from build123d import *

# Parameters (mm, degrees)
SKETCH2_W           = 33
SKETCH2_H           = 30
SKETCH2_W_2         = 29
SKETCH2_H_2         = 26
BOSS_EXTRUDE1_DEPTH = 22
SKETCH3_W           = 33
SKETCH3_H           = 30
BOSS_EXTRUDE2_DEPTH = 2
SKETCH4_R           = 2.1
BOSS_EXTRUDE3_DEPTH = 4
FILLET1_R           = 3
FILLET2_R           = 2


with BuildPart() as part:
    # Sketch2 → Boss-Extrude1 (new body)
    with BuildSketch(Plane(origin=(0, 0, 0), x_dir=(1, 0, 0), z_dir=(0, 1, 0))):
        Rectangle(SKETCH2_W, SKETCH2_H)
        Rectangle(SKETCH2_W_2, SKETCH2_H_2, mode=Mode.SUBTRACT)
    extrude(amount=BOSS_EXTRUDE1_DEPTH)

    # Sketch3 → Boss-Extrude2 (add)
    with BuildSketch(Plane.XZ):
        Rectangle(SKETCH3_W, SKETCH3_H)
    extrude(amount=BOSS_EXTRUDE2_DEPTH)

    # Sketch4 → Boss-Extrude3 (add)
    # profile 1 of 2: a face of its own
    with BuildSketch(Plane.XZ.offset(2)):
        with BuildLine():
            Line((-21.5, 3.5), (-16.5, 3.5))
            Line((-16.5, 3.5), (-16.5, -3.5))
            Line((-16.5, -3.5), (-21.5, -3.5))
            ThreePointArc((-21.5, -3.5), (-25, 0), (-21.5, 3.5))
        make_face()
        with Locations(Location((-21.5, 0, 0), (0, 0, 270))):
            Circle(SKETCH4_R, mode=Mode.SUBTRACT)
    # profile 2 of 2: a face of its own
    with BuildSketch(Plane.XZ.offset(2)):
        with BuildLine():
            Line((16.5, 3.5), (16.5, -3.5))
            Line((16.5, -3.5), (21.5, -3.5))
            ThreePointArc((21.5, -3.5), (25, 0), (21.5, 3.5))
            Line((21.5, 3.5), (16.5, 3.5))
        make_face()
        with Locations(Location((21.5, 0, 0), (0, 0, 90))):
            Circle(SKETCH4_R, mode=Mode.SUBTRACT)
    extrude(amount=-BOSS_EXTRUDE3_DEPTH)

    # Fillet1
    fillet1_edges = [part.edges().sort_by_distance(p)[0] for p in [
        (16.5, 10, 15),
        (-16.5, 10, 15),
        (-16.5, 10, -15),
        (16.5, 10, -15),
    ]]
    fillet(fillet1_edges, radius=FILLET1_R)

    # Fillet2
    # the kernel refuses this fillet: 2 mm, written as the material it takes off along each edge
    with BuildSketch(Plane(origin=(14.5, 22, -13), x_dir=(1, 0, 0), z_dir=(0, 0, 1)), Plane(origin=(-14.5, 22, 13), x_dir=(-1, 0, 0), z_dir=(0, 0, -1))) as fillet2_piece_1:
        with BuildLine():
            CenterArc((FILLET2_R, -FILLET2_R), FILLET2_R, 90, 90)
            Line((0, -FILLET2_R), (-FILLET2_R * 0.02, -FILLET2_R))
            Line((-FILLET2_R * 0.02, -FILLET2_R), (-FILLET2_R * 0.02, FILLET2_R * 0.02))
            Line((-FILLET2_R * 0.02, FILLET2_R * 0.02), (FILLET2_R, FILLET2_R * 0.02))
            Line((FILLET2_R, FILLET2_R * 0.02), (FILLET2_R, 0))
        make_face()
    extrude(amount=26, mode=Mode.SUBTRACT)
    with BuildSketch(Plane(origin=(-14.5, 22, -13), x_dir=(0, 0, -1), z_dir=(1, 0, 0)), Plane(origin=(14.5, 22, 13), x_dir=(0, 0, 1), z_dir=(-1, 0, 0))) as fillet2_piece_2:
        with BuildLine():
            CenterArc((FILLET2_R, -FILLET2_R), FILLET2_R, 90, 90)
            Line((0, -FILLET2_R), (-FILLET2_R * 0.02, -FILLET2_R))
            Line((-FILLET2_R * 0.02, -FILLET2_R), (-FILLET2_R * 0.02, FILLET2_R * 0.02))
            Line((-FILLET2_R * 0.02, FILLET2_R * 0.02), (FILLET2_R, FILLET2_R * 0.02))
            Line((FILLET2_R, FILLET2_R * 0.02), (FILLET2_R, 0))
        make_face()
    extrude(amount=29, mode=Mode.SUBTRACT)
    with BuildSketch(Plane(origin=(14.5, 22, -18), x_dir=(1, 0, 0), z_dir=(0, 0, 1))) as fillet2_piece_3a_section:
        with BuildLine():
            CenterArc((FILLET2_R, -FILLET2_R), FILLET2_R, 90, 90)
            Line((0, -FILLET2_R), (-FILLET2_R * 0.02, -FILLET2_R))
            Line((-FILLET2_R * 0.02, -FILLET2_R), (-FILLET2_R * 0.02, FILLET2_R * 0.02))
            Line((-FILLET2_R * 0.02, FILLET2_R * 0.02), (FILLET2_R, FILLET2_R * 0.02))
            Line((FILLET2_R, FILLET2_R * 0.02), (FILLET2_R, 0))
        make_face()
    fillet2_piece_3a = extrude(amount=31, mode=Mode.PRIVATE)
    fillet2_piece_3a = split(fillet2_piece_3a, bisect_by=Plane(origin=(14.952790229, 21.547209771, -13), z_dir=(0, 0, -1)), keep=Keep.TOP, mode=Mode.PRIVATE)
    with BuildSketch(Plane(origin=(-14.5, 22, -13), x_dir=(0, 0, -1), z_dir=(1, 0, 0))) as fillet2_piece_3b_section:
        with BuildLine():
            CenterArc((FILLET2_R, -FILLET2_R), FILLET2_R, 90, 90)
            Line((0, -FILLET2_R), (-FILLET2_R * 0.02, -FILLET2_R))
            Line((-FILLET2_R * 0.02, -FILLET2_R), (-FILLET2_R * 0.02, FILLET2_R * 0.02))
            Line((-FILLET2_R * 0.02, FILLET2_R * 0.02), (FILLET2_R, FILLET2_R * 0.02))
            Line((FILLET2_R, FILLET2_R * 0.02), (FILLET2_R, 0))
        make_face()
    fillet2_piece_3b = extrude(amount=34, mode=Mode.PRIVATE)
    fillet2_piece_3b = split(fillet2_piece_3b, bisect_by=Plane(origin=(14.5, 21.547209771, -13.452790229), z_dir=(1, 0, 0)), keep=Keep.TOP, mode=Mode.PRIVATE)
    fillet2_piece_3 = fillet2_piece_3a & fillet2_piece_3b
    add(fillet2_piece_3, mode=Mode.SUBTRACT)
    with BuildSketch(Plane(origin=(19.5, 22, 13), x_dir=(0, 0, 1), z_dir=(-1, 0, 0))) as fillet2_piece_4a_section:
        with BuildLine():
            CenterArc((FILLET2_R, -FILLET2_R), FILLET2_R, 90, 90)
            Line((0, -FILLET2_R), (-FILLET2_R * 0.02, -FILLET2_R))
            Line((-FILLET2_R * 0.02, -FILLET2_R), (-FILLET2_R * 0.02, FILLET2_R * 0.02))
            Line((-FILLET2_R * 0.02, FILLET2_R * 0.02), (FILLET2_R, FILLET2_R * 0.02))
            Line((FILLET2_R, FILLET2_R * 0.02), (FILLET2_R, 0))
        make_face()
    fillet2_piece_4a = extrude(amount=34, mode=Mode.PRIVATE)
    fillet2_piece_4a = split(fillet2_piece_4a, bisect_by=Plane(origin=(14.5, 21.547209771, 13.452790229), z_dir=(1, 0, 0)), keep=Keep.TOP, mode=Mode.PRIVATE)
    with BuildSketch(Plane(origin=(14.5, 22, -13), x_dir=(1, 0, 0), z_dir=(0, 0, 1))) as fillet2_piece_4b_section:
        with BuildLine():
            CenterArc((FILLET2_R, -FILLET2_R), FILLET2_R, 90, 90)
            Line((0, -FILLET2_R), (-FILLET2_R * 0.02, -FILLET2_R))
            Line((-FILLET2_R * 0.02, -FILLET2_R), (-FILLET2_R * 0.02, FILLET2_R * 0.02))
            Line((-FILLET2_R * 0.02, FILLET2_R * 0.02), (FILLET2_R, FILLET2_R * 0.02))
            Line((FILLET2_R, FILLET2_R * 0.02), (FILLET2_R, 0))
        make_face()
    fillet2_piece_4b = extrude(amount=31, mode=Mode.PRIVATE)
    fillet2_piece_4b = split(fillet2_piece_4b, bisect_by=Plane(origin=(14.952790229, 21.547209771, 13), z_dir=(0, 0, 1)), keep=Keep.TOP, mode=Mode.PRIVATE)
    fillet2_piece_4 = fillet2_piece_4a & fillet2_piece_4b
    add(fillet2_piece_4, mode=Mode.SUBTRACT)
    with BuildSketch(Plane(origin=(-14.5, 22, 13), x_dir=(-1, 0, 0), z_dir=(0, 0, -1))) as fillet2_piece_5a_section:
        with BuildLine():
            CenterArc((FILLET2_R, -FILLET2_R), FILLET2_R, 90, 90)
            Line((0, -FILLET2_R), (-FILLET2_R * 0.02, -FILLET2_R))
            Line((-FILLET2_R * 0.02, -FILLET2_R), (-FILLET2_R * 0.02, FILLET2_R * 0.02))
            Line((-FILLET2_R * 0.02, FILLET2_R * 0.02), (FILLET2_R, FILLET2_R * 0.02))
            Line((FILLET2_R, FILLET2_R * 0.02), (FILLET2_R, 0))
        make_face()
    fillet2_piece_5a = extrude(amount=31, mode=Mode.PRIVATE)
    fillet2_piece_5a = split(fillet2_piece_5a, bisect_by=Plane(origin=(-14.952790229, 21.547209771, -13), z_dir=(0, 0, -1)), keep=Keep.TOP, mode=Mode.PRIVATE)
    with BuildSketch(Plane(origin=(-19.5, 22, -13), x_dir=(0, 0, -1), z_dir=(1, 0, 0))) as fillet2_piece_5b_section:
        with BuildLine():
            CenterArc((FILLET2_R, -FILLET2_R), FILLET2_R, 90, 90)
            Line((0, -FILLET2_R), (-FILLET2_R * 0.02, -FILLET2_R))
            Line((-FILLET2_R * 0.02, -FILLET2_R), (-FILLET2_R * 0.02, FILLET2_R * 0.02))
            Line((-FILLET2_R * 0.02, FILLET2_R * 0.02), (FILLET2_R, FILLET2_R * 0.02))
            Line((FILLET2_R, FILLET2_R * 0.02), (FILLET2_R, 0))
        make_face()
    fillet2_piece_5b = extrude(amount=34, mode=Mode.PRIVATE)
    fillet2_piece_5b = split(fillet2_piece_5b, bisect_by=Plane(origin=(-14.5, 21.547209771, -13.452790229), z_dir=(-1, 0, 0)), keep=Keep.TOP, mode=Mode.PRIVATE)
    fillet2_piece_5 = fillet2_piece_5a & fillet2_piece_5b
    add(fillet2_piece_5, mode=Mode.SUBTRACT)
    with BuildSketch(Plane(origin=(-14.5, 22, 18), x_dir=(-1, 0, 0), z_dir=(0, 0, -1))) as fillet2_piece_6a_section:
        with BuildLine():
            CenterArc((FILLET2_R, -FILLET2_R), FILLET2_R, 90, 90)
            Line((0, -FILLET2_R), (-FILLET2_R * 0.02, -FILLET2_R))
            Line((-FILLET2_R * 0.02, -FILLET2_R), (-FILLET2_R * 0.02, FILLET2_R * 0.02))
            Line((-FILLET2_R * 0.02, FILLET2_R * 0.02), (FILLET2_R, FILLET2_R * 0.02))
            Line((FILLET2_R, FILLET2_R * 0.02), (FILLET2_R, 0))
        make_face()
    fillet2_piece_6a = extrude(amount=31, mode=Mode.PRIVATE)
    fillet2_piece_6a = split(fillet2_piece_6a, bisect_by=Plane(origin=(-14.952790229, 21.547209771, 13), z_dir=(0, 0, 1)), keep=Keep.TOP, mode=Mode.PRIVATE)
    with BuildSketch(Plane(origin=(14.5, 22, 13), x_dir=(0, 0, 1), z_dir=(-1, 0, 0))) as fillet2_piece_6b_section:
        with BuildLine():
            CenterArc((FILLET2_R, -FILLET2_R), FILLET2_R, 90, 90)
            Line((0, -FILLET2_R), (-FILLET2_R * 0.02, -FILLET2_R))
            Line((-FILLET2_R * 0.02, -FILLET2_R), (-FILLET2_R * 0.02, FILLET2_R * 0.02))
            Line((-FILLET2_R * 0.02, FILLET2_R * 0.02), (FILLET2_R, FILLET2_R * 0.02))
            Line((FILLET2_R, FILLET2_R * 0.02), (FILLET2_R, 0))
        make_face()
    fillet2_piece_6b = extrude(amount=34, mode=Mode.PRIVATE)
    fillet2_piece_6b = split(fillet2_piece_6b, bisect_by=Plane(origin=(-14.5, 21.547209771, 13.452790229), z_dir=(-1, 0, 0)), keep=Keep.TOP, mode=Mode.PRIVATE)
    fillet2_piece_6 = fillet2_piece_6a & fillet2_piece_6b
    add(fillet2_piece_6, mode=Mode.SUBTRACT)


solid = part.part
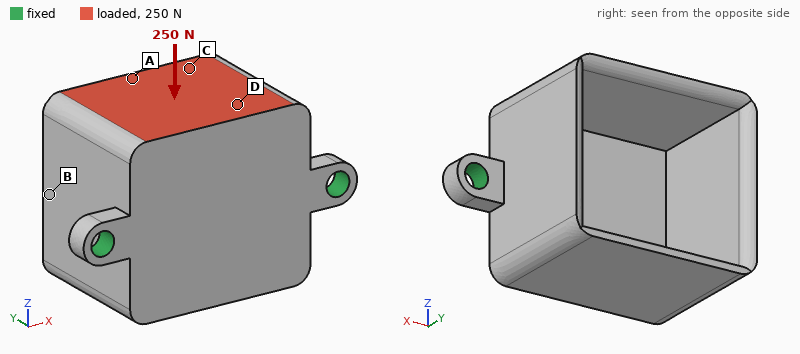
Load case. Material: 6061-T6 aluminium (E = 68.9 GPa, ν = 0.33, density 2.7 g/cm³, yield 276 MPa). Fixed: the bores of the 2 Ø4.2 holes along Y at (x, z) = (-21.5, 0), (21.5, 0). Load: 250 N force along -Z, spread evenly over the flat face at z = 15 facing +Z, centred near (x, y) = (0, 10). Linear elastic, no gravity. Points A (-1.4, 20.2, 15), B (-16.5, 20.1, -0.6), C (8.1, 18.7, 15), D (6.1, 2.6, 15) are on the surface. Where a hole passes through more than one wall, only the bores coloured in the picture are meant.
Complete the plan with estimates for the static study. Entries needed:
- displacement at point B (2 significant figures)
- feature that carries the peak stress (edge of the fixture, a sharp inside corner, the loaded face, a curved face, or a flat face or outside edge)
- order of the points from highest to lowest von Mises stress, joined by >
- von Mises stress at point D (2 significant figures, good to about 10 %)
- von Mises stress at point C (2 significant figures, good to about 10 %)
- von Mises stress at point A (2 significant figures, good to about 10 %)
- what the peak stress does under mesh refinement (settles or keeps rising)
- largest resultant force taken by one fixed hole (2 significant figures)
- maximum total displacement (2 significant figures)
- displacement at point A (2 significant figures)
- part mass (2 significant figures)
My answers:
46 µm
edge of the fixture
A > C > D > B
13 MPa
19 MPa
28 MPa
keeps rising
130 N
99 µm
91 µm
19 g
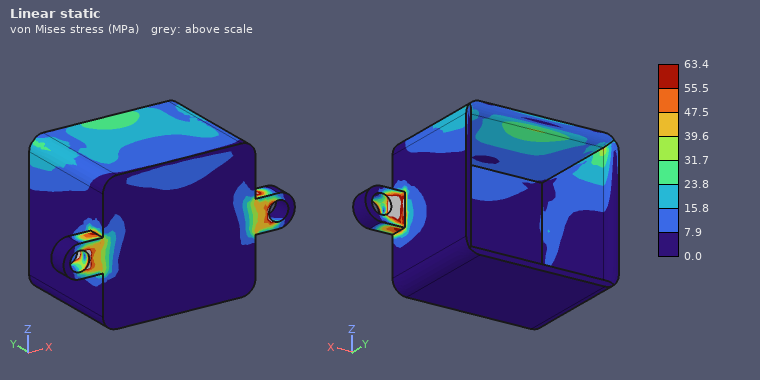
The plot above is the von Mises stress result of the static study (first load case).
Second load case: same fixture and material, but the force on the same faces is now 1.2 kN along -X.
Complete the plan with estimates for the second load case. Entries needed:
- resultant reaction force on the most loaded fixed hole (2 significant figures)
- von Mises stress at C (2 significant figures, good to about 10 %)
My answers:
840 N
29 MPa
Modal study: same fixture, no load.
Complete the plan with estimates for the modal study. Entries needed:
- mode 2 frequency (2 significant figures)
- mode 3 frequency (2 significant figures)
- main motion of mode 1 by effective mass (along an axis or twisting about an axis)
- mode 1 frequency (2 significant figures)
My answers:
4800 Hz
7500 Hz
along Z
2600 Hz
